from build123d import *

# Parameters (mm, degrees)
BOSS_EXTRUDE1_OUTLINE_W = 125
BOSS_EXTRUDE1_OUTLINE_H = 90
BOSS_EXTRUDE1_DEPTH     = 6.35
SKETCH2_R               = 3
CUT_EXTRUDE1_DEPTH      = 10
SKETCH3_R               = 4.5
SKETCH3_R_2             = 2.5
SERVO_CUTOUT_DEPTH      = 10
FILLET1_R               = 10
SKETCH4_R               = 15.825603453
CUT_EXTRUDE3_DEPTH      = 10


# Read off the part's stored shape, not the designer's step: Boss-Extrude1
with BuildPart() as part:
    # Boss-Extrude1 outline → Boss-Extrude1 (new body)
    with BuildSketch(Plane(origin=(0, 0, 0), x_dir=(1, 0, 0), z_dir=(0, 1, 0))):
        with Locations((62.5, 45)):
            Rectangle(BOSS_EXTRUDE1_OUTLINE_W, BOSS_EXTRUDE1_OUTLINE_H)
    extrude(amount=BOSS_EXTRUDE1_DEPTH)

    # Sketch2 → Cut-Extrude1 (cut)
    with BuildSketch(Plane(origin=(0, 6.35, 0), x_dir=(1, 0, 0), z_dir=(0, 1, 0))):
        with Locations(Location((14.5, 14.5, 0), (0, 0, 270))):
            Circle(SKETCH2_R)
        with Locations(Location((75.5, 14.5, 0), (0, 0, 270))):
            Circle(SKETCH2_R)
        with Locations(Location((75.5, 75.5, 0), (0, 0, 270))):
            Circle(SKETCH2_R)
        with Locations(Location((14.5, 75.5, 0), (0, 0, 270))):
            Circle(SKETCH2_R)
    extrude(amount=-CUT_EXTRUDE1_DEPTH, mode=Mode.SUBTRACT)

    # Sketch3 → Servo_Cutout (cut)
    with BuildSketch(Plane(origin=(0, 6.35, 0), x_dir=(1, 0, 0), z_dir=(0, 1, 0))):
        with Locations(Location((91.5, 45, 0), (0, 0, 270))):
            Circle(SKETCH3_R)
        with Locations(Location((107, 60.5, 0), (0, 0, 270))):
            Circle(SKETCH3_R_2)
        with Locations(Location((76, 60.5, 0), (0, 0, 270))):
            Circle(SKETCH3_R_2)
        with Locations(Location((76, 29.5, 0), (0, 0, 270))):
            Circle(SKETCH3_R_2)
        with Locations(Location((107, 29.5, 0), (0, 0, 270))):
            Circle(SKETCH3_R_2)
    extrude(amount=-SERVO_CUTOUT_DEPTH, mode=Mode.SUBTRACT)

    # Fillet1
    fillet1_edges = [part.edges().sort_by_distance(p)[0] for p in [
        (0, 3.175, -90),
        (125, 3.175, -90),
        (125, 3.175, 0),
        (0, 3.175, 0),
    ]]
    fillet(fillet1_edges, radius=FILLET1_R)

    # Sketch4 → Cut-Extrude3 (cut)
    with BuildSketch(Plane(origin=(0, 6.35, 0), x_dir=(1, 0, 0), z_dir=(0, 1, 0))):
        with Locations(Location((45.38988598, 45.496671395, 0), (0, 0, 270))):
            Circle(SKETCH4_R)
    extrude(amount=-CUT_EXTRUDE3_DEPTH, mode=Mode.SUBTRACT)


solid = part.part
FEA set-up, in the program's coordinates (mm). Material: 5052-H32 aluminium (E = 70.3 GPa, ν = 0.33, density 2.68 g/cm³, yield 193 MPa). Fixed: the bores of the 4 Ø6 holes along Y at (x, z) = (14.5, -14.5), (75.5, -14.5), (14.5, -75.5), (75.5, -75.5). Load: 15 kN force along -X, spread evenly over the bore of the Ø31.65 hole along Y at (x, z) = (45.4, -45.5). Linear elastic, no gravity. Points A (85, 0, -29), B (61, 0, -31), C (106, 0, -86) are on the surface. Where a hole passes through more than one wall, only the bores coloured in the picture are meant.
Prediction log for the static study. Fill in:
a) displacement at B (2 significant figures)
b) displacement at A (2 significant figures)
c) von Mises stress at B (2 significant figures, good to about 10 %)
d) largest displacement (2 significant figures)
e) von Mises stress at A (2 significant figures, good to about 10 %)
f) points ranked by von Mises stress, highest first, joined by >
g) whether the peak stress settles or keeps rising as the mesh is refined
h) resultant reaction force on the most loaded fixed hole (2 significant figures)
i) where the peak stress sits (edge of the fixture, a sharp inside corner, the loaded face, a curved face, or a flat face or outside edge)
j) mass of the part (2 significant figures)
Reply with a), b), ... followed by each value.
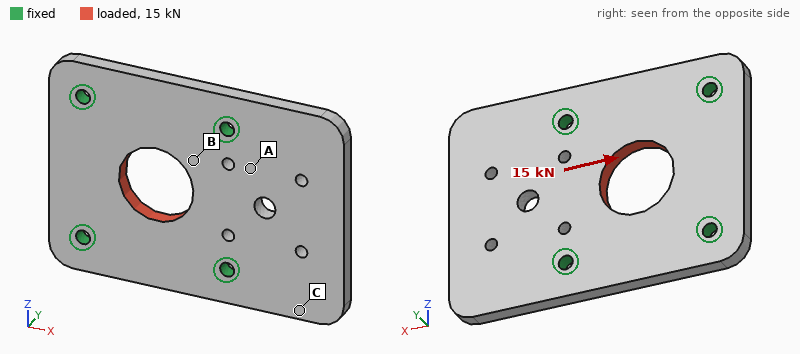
a) 10 µm
b) 6.1 µm
c) 23 MPa
d) 18 µm
e) 12 MPa
f) B > A > C
g) keeps rising
h) 4.1 kN
i) edge of the fixture
j) 170 g
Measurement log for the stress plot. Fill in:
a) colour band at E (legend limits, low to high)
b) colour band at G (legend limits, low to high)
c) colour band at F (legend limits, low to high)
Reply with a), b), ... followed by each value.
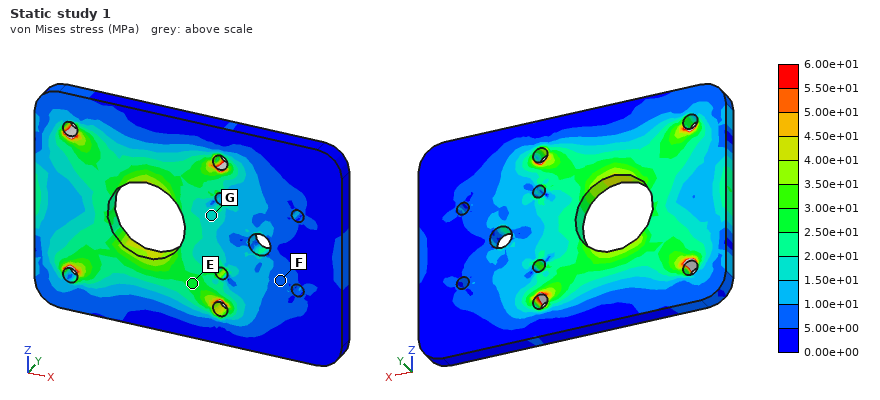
a) 2.50e+01 to 3.00e+01 MPa
b) 1.50e+01 to 2.00e+01 MPa
c) 5.00e+00 to 1.00e+01 MPa
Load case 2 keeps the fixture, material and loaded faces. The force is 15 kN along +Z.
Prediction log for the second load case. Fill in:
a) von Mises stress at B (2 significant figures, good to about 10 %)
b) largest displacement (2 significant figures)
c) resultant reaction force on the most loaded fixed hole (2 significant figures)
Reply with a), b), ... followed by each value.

a) 25 MPa
b) 18 µm
c) 4.0 kN
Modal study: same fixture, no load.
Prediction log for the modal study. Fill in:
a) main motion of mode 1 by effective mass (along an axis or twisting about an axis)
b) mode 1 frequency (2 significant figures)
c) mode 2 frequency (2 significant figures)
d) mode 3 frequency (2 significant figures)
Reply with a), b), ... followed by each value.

a) along Y
b) 1900 Hz
c) 3400 Hz
d) 6200 Hz
